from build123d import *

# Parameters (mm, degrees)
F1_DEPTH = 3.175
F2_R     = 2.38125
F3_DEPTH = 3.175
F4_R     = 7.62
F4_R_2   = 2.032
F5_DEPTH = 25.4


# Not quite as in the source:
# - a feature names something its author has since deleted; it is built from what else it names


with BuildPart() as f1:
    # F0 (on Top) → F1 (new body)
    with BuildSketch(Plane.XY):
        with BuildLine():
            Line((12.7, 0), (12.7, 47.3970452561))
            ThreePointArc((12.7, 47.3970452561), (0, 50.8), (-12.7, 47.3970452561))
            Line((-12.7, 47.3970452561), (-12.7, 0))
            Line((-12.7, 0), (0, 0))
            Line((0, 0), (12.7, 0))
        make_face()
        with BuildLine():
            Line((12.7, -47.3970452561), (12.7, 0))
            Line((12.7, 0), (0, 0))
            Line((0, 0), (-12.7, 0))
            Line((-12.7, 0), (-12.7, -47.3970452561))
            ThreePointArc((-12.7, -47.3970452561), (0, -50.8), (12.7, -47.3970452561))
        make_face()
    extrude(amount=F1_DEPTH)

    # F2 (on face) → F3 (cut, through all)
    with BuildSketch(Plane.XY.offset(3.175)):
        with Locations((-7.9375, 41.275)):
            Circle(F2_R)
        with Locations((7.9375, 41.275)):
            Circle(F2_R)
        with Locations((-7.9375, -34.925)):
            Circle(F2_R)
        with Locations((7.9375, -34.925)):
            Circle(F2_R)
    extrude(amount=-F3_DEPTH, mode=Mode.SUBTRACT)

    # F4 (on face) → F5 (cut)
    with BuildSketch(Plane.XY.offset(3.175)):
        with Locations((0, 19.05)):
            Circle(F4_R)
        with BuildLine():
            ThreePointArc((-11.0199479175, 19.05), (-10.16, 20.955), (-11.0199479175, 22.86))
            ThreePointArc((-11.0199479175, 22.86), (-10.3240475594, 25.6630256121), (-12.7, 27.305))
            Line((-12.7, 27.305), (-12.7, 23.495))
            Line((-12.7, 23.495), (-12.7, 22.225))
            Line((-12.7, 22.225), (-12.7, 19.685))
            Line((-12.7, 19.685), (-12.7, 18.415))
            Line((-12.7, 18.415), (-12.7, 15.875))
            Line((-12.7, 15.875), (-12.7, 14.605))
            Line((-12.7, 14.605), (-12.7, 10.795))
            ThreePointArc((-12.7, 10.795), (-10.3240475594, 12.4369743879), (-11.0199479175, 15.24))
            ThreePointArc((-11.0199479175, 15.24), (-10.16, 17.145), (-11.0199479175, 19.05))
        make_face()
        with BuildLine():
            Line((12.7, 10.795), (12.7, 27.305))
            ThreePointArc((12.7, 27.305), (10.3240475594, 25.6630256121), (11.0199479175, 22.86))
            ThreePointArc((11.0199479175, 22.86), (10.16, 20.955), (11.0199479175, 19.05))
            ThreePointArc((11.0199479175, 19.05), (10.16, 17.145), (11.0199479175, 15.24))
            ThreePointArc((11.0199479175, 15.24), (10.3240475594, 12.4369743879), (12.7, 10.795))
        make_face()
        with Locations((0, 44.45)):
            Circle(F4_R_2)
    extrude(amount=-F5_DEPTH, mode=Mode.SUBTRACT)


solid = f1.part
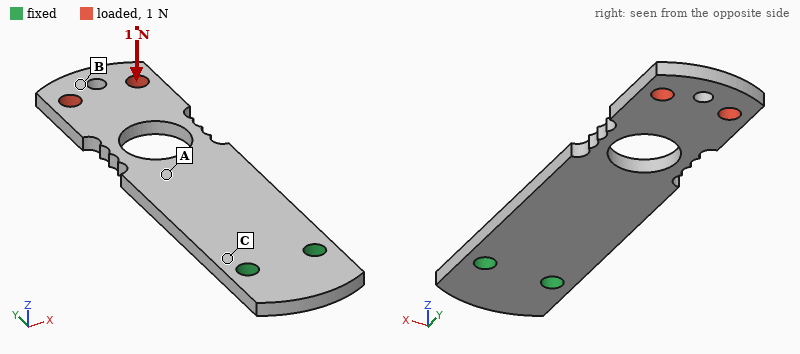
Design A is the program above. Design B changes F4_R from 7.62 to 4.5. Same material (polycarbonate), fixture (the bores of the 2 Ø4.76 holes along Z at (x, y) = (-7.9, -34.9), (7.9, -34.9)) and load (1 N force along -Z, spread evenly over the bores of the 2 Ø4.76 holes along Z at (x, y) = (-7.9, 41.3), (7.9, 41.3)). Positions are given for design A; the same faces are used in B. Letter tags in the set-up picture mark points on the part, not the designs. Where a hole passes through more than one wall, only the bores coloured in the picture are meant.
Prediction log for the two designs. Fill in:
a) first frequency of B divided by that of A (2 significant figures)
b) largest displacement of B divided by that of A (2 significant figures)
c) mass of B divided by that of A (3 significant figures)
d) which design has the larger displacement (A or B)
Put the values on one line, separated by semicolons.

1.0; 0.89; 1.05; A
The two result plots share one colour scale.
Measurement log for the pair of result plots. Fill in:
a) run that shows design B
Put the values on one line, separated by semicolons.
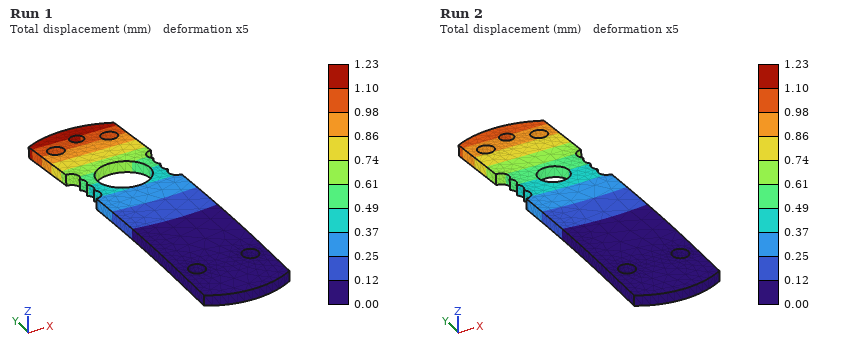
Run 2
